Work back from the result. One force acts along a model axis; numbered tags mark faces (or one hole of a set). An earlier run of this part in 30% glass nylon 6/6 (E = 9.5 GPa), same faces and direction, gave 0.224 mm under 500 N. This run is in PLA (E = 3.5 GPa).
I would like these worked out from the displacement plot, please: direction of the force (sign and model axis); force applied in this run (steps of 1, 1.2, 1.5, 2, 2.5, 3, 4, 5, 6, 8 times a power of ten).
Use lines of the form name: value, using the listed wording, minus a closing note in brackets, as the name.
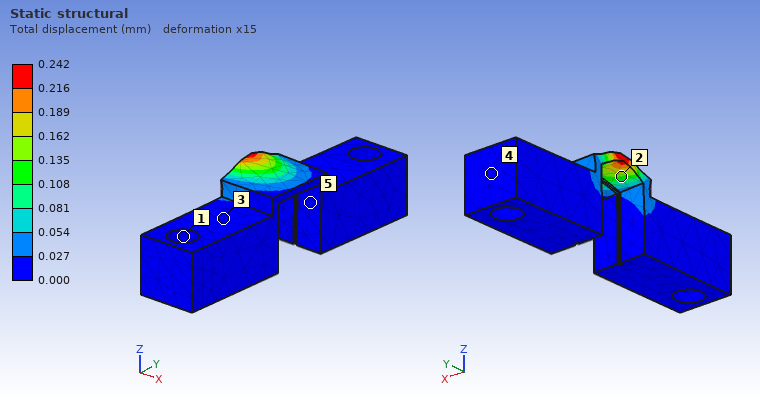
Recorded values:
direction of the force: +Z
force applied in this run: 200 N
